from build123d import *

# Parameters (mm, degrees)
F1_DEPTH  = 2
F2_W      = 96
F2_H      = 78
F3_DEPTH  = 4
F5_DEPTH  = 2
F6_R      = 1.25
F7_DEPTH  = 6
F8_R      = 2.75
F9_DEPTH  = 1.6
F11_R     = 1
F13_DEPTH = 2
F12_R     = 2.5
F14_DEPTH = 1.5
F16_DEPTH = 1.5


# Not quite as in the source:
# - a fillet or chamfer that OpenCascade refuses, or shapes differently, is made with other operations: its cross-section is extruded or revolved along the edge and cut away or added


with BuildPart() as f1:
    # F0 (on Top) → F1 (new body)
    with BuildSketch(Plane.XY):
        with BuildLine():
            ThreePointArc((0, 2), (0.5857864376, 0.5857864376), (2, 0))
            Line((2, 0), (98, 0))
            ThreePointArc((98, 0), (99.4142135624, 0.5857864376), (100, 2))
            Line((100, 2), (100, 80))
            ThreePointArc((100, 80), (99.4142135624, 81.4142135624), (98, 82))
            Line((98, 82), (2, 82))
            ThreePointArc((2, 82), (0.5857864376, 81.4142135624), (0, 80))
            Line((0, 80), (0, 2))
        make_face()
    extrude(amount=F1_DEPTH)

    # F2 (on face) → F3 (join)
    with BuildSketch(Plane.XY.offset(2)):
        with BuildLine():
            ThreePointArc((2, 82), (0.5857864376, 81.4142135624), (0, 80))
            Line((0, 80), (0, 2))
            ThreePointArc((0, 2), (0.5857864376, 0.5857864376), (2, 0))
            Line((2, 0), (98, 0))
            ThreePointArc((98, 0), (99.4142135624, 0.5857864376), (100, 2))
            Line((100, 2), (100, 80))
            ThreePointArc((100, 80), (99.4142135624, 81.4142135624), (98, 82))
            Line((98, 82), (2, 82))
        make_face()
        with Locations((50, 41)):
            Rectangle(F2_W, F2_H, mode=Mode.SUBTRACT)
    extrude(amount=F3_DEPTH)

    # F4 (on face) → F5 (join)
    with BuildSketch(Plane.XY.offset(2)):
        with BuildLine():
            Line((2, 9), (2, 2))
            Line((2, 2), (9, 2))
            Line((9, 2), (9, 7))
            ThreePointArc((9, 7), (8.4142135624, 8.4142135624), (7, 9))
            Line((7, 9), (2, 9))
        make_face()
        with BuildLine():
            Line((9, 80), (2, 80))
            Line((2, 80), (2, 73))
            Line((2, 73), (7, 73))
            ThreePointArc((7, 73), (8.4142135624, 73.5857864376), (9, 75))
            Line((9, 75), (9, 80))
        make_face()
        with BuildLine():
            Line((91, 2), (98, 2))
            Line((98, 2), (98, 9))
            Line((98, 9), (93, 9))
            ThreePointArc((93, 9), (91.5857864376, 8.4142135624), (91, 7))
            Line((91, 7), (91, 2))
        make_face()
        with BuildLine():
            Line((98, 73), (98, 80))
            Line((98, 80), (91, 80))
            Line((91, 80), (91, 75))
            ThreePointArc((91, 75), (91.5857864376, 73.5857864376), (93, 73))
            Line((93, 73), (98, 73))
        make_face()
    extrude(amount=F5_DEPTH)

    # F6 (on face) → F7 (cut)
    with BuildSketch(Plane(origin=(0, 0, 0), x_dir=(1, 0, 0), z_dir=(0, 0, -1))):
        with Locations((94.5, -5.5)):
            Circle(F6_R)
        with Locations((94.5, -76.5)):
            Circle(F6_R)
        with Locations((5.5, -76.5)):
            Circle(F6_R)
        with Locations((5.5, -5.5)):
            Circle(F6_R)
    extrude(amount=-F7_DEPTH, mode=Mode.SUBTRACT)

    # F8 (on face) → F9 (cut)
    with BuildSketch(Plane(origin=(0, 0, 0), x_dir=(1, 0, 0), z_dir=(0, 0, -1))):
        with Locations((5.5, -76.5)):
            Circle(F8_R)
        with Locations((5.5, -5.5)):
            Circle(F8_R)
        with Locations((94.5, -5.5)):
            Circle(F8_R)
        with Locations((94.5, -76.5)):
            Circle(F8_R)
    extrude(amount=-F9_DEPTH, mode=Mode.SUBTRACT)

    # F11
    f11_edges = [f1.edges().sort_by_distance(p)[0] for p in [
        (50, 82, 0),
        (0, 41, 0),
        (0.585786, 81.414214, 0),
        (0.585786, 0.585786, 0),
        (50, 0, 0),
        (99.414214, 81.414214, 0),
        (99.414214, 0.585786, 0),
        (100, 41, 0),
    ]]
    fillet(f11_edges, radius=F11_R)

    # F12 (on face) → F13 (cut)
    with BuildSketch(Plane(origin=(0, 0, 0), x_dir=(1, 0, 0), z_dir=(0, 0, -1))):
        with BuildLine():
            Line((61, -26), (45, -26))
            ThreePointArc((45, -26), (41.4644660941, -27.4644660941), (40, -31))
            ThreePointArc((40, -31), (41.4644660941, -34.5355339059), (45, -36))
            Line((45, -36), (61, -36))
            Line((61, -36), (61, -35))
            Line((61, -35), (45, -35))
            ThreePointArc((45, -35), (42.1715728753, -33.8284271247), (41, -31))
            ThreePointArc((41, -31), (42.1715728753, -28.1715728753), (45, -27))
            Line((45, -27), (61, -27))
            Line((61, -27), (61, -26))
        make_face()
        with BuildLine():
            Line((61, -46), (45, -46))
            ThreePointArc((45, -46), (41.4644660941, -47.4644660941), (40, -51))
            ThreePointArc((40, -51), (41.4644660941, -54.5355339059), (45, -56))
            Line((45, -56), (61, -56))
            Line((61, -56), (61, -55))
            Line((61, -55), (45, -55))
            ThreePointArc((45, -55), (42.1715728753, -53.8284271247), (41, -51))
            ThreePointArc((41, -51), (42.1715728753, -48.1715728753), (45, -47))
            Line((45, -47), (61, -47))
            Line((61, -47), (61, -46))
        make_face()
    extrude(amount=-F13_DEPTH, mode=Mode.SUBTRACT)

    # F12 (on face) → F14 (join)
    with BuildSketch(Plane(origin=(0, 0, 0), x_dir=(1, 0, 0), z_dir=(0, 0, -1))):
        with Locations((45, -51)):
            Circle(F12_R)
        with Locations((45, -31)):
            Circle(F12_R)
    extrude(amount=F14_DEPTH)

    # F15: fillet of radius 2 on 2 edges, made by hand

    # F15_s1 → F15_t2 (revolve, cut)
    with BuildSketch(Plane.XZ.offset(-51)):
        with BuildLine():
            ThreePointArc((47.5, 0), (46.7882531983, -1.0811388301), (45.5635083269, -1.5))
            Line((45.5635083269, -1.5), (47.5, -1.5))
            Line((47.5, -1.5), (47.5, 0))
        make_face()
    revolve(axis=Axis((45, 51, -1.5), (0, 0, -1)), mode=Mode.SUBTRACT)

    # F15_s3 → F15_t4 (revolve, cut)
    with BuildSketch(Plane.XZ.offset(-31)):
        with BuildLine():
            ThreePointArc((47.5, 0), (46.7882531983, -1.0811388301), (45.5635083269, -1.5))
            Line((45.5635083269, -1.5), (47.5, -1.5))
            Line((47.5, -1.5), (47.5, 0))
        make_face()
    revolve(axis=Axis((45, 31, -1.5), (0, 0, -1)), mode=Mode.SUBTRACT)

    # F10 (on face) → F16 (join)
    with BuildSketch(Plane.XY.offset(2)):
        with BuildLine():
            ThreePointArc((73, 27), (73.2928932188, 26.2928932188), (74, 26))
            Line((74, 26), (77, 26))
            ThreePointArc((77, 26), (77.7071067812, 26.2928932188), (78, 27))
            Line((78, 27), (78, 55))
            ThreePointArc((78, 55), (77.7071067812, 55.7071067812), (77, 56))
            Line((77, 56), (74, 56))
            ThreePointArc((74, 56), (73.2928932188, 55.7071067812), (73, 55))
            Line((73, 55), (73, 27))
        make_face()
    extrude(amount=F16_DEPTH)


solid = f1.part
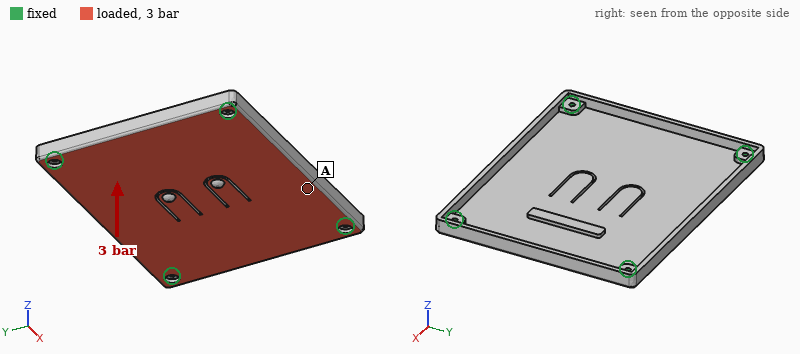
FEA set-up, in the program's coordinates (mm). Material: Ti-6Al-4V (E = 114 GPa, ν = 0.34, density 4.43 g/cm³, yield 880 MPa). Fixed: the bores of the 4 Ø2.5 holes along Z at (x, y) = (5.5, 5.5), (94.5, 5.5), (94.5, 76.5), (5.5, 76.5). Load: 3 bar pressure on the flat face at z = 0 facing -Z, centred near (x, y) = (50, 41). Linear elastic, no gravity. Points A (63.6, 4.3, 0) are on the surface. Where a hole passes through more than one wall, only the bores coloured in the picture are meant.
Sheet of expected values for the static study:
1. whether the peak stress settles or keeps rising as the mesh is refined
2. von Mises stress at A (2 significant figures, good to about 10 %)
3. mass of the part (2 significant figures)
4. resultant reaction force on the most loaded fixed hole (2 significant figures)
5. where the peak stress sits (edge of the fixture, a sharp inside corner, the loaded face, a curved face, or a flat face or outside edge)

keeps rising
87 MPa
86 g
1.3 kN
edge of the fixture
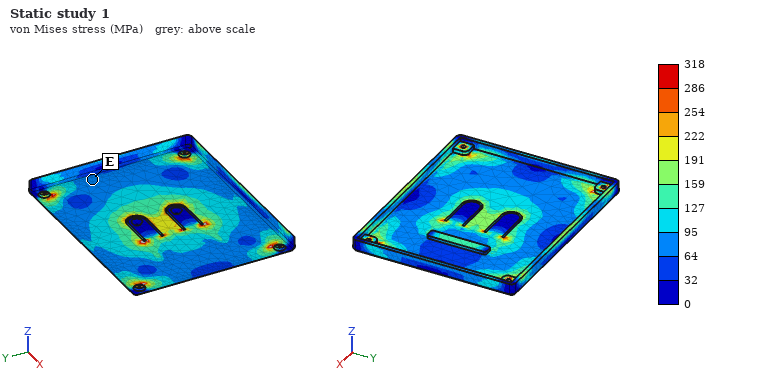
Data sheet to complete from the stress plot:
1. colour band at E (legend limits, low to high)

64 to 95 MPa
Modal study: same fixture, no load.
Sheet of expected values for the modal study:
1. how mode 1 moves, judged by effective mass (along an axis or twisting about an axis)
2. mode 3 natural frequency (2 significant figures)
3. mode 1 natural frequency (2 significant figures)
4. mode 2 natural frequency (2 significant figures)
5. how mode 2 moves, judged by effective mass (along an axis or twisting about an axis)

along Z
2600 Hz
1100 Hz
2200 Hz
twisting about X
